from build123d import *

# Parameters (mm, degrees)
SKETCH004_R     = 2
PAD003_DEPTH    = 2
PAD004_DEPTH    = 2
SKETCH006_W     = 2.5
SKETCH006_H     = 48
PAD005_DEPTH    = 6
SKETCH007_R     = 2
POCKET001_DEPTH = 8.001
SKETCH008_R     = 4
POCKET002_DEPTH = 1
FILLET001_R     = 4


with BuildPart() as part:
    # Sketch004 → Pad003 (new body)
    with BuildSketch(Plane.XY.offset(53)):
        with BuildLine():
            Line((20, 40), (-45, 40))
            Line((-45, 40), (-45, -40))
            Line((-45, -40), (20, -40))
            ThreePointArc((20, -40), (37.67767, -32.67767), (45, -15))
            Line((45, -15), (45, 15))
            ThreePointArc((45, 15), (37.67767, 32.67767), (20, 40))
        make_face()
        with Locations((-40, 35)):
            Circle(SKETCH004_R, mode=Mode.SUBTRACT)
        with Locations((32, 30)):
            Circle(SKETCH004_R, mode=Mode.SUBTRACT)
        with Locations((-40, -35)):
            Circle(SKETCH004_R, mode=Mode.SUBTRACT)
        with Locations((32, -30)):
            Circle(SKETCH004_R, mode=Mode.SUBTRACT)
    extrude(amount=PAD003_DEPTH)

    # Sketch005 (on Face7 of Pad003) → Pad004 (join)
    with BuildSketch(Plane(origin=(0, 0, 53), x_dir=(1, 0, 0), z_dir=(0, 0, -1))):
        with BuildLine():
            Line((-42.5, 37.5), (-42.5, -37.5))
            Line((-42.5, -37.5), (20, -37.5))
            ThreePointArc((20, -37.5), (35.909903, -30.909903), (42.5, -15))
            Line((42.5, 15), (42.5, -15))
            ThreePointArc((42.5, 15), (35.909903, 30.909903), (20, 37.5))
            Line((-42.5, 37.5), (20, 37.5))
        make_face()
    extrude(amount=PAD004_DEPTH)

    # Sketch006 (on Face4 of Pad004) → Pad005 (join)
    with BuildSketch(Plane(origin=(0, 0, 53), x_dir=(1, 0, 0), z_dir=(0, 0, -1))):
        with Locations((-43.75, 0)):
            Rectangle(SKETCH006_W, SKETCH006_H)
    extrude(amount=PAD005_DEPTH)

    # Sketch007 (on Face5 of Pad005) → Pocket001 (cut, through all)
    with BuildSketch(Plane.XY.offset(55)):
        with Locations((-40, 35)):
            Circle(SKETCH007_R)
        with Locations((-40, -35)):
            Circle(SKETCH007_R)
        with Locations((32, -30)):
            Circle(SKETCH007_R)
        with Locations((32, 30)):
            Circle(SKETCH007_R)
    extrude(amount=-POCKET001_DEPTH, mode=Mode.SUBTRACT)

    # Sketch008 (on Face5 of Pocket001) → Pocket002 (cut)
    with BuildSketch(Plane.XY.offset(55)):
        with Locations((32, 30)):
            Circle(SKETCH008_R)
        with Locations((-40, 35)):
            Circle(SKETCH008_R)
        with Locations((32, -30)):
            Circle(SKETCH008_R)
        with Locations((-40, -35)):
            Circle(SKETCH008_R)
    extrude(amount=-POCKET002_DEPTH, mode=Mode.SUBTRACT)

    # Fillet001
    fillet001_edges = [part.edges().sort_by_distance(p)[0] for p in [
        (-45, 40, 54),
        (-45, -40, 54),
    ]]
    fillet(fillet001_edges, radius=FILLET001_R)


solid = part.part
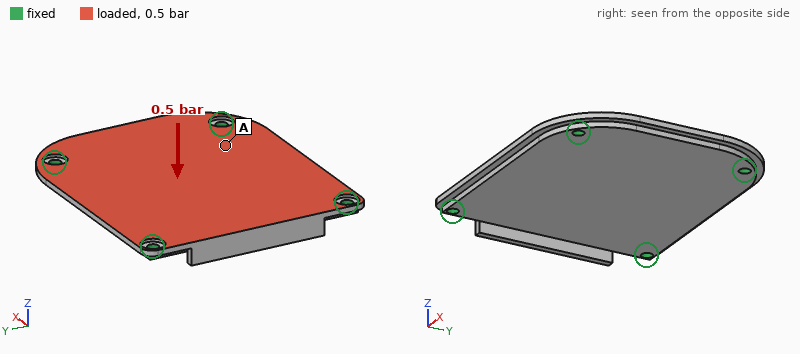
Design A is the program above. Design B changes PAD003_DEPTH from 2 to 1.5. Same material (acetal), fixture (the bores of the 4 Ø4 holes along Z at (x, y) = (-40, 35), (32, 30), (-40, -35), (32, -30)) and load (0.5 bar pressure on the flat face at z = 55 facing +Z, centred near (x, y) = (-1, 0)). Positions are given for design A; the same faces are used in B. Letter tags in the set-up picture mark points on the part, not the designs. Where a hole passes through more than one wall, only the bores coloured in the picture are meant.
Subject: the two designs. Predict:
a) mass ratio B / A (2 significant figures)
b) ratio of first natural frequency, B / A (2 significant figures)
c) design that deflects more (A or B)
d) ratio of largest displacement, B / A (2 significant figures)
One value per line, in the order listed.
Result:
0.87
0.92
B
1.3
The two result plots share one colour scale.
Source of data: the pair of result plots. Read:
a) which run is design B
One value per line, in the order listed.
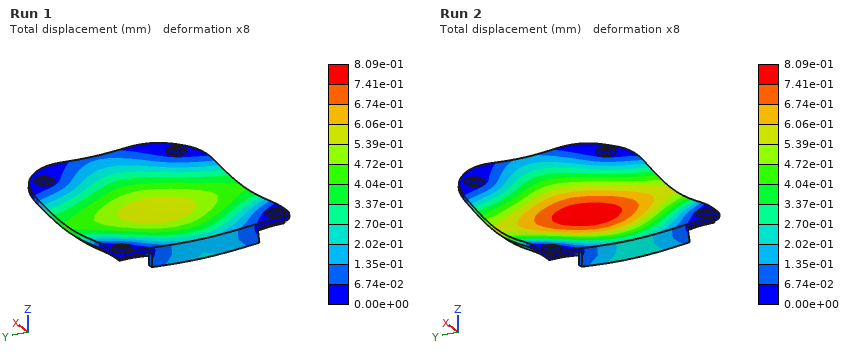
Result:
Run 2
